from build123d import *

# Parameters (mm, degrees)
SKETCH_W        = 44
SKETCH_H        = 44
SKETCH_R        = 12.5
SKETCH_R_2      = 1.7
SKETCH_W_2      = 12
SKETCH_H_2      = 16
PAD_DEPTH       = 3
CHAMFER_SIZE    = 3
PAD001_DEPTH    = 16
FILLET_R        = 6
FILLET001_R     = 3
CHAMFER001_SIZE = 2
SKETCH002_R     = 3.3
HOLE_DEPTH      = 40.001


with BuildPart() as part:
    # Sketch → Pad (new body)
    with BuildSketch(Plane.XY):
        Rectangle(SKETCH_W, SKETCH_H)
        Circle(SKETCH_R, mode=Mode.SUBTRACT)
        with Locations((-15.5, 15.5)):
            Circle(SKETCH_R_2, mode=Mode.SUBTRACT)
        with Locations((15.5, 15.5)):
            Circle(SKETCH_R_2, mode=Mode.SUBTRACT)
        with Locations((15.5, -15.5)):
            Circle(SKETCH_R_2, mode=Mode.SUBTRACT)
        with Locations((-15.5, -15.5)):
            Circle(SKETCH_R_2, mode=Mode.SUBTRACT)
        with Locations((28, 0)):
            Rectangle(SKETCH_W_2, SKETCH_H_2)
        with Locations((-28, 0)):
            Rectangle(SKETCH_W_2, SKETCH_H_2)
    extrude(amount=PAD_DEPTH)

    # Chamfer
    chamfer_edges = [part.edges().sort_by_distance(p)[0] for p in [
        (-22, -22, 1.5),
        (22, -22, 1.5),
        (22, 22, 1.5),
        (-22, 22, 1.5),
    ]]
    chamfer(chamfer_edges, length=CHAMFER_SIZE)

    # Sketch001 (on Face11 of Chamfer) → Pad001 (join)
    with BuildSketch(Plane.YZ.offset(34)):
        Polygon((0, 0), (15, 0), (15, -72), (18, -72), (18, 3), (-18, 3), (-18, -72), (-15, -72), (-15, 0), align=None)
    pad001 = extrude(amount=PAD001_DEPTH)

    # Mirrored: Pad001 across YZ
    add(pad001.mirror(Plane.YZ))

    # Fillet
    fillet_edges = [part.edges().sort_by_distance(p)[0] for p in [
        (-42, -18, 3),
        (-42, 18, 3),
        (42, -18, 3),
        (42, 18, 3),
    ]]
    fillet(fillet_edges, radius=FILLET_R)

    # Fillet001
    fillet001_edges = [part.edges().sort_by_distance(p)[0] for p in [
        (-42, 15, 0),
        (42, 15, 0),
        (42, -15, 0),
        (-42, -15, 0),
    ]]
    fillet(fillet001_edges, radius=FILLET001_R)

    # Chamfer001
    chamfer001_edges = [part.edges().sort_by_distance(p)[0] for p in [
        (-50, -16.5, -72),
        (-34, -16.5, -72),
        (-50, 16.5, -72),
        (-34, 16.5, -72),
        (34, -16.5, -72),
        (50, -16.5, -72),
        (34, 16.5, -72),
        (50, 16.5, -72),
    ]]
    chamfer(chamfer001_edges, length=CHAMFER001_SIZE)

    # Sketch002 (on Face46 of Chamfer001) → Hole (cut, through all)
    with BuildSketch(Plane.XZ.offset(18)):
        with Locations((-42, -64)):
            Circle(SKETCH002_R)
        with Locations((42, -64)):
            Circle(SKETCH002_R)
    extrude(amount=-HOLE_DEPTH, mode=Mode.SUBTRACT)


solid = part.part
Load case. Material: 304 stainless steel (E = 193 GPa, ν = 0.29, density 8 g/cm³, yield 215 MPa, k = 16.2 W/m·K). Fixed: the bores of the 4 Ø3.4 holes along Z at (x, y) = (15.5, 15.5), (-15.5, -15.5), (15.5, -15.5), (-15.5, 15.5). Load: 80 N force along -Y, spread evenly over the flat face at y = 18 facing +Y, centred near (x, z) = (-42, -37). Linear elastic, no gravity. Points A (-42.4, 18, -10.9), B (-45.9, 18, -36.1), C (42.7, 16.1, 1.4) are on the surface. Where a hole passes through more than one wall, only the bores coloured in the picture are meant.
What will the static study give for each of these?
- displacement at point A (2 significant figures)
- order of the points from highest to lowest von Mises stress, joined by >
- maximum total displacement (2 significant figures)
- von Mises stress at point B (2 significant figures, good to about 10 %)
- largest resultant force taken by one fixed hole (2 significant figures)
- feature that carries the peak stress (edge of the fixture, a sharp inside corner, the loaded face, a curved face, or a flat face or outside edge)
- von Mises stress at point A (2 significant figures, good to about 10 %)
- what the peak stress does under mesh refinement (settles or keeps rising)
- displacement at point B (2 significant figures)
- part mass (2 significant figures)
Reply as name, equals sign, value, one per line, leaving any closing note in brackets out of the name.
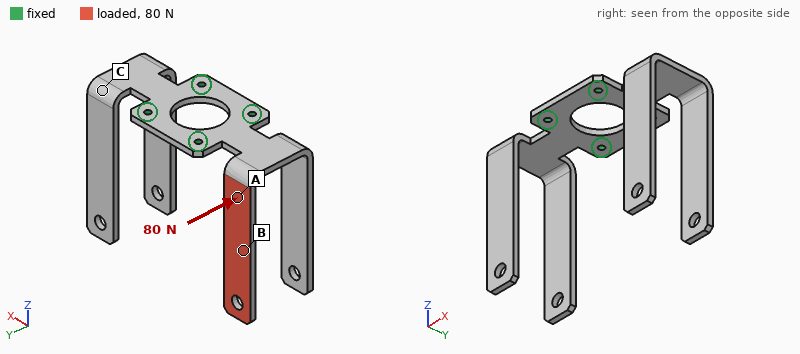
displacement at point A = 0.21 mm
order of the points from highest to lowest von Mises stress, joined by > = A > B > C
maximum total displacement = 1.3 mm
von Mises stress at point B = 29 MPa
largest resultant force taken by one fixed hole = 160 N
feature that carries the peak stress = a sharp inside corner
von Mises stress at point A = 81 MPa
what the peak stress does under mesh refinement = keeps rising
displacement at point B = 0.62 mm
part mass = 170 g
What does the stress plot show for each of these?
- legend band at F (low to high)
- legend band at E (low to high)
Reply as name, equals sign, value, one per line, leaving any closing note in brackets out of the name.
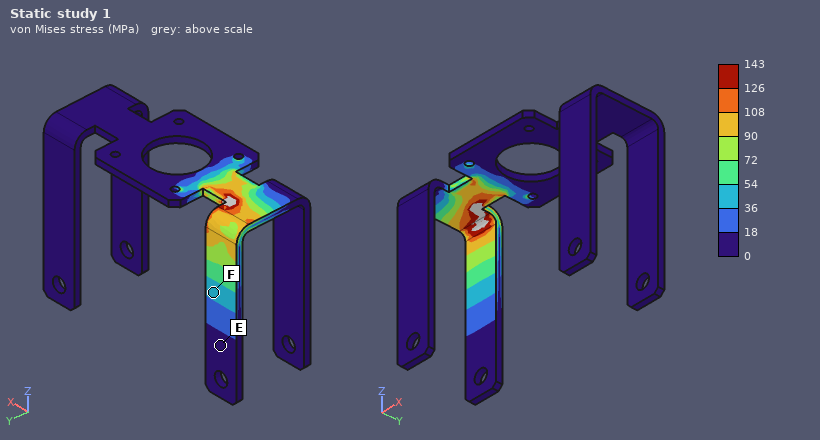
legend band at F = 36 to 54 MPa
legend band at E = 0 to 18 MPa
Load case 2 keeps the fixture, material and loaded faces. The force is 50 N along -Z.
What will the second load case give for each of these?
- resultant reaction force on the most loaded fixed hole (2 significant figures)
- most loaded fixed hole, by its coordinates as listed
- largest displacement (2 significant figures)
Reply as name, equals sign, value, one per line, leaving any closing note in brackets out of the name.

resultant reaction force on the most loaded fixed hole = 71 N
most loaded fixed hole, by its coordinates as listed = (-15.5, 15.5)
largest displacement = 0.31 mm
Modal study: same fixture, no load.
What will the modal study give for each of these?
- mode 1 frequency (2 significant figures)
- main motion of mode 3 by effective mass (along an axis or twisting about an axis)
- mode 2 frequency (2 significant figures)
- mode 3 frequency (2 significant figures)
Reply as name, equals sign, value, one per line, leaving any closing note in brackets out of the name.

mode 1 frequency = 250 Hz
main motion of mode 3 by effective mass = along Y
mode 2 frequency = 250 Hz
mode 3 frequency = 260 Hz
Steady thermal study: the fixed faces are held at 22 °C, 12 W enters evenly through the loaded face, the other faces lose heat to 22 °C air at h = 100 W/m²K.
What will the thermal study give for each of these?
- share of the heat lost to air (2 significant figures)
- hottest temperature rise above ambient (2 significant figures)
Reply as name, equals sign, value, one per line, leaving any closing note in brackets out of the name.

share of the heat lost to air = 99 %
hottest temperature rise above ambient = 74 K
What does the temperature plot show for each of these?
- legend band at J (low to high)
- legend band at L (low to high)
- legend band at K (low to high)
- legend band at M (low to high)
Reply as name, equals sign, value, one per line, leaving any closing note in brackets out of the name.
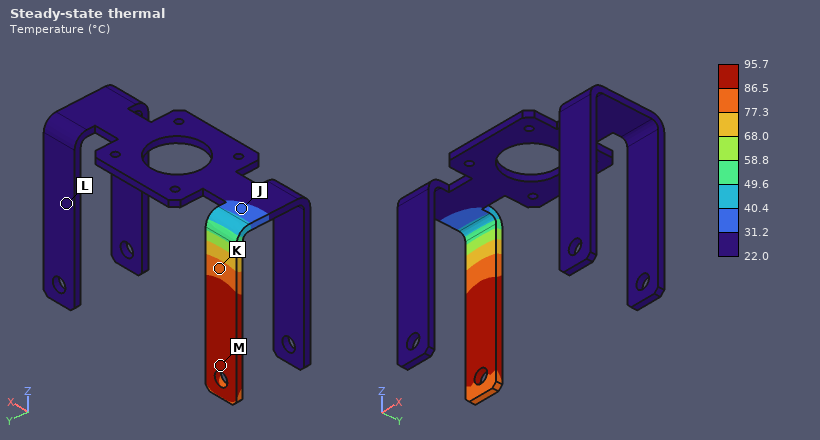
legend band at J = 31.2 to 40.4 °C
legend band at L = 22.0 to 31.2 °C
legend band at K = 77.3 to 86.5 °C
legend band at M = 86.5 to 95.7 °C
